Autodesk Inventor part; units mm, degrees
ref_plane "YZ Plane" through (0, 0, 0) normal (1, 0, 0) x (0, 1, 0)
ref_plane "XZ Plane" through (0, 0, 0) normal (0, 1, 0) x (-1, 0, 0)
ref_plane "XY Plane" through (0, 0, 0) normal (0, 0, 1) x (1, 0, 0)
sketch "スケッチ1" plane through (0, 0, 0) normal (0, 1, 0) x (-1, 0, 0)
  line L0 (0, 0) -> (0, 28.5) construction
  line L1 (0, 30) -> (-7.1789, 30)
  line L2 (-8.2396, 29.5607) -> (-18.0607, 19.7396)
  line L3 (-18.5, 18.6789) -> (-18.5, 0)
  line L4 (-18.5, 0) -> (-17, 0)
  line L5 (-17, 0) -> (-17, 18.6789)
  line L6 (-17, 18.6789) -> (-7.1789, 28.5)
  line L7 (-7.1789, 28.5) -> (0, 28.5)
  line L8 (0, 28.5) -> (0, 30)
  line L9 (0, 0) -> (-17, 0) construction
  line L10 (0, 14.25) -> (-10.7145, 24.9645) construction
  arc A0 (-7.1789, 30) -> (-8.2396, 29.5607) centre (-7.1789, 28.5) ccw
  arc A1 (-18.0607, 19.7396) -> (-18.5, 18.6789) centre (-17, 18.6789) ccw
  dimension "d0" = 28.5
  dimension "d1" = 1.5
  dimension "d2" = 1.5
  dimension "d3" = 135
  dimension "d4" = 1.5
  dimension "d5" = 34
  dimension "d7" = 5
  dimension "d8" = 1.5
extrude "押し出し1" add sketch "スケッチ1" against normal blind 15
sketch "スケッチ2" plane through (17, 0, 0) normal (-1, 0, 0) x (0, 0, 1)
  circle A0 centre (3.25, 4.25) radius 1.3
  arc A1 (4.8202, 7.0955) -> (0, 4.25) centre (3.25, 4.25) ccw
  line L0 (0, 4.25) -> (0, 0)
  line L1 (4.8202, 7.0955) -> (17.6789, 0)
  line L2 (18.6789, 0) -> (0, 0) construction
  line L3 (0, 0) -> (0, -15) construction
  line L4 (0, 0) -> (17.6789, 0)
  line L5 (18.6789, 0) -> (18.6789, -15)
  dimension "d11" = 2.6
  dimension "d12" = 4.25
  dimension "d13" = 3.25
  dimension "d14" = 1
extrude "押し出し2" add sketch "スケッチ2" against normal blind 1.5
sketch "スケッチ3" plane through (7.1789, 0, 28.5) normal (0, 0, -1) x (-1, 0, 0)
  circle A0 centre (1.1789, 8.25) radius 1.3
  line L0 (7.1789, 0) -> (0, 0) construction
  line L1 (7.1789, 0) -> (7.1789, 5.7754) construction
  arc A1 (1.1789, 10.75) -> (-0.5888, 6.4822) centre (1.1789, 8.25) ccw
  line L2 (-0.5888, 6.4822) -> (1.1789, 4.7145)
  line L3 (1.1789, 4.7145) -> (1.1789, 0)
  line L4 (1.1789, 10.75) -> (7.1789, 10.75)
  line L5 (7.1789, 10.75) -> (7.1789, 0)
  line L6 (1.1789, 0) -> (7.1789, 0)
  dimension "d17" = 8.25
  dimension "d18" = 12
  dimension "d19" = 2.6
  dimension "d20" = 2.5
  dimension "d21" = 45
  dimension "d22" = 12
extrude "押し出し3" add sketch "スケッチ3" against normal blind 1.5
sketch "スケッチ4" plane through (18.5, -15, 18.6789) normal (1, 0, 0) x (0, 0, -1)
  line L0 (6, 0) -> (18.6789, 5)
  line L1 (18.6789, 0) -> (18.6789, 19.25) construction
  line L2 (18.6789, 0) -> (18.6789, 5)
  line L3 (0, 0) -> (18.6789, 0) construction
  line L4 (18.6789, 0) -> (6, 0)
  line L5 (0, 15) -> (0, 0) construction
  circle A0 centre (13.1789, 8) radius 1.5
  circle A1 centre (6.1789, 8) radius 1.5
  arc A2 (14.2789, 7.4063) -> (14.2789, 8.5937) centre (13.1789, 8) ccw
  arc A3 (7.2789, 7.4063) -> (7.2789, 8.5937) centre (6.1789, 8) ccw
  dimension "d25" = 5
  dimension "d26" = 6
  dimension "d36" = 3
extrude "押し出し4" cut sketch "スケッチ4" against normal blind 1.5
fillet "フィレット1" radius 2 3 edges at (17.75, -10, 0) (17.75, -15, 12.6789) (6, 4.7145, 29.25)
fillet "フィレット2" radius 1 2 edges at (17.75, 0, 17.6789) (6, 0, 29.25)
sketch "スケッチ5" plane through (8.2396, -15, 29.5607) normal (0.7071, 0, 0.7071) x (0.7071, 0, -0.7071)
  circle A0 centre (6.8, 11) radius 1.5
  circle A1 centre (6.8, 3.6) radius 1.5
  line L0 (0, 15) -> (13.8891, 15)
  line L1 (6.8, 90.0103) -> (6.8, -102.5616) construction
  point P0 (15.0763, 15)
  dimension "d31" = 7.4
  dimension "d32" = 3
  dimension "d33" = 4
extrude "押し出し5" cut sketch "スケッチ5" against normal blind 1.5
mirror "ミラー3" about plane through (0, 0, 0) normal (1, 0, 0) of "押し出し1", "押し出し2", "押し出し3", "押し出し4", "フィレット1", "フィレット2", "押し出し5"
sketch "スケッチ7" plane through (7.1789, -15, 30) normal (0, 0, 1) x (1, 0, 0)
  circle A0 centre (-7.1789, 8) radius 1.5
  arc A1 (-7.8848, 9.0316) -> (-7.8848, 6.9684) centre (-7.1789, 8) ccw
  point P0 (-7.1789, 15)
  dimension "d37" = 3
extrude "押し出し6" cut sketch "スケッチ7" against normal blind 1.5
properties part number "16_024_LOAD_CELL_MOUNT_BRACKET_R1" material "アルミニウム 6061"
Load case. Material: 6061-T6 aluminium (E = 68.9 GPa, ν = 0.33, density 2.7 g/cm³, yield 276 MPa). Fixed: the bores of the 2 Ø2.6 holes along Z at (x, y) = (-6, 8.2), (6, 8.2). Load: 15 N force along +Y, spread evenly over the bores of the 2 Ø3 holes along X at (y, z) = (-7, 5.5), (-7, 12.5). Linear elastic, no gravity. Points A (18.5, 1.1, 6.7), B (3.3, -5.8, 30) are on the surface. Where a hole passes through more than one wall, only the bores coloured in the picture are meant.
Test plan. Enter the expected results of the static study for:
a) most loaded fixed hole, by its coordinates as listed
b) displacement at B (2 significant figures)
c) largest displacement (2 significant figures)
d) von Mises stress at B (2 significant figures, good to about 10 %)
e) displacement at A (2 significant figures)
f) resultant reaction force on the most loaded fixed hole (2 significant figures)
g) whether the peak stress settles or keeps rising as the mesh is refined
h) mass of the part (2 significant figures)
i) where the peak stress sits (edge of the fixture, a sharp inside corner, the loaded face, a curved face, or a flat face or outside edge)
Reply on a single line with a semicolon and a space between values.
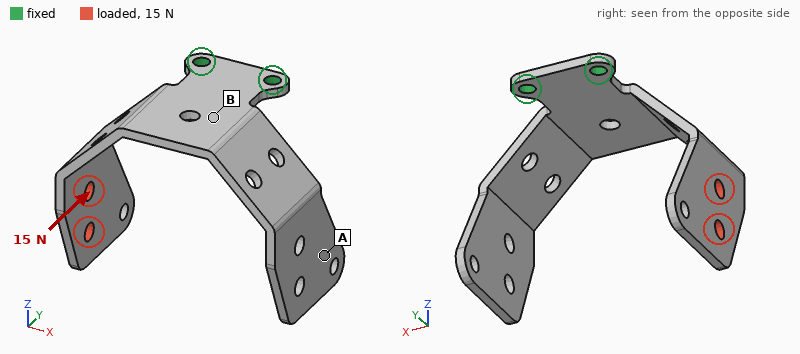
(-6, 8.2); 0.11 mm; 0.59 mm; 19 MPa; 0.28 mm; 31 N; keeps rising; 5.6 g; a sharp inside corner
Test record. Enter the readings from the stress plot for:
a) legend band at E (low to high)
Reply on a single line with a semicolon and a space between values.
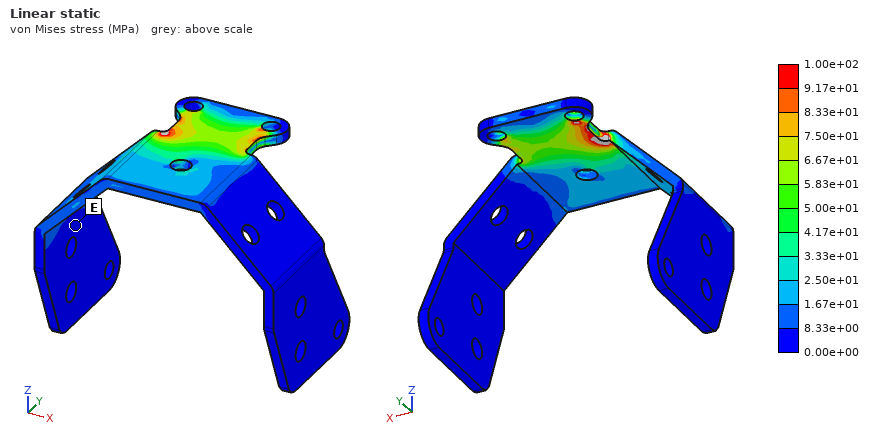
0.00e+00 to 8.33e+00 MPa
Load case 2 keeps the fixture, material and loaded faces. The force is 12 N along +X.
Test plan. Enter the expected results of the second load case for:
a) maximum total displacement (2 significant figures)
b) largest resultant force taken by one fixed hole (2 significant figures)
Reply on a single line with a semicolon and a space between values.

0.60 mm; 28 N
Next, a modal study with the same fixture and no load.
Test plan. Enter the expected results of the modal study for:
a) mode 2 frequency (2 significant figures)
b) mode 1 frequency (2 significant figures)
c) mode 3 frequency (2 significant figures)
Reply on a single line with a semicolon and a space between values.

570 Hz; 570 Hz; 790 Hz
